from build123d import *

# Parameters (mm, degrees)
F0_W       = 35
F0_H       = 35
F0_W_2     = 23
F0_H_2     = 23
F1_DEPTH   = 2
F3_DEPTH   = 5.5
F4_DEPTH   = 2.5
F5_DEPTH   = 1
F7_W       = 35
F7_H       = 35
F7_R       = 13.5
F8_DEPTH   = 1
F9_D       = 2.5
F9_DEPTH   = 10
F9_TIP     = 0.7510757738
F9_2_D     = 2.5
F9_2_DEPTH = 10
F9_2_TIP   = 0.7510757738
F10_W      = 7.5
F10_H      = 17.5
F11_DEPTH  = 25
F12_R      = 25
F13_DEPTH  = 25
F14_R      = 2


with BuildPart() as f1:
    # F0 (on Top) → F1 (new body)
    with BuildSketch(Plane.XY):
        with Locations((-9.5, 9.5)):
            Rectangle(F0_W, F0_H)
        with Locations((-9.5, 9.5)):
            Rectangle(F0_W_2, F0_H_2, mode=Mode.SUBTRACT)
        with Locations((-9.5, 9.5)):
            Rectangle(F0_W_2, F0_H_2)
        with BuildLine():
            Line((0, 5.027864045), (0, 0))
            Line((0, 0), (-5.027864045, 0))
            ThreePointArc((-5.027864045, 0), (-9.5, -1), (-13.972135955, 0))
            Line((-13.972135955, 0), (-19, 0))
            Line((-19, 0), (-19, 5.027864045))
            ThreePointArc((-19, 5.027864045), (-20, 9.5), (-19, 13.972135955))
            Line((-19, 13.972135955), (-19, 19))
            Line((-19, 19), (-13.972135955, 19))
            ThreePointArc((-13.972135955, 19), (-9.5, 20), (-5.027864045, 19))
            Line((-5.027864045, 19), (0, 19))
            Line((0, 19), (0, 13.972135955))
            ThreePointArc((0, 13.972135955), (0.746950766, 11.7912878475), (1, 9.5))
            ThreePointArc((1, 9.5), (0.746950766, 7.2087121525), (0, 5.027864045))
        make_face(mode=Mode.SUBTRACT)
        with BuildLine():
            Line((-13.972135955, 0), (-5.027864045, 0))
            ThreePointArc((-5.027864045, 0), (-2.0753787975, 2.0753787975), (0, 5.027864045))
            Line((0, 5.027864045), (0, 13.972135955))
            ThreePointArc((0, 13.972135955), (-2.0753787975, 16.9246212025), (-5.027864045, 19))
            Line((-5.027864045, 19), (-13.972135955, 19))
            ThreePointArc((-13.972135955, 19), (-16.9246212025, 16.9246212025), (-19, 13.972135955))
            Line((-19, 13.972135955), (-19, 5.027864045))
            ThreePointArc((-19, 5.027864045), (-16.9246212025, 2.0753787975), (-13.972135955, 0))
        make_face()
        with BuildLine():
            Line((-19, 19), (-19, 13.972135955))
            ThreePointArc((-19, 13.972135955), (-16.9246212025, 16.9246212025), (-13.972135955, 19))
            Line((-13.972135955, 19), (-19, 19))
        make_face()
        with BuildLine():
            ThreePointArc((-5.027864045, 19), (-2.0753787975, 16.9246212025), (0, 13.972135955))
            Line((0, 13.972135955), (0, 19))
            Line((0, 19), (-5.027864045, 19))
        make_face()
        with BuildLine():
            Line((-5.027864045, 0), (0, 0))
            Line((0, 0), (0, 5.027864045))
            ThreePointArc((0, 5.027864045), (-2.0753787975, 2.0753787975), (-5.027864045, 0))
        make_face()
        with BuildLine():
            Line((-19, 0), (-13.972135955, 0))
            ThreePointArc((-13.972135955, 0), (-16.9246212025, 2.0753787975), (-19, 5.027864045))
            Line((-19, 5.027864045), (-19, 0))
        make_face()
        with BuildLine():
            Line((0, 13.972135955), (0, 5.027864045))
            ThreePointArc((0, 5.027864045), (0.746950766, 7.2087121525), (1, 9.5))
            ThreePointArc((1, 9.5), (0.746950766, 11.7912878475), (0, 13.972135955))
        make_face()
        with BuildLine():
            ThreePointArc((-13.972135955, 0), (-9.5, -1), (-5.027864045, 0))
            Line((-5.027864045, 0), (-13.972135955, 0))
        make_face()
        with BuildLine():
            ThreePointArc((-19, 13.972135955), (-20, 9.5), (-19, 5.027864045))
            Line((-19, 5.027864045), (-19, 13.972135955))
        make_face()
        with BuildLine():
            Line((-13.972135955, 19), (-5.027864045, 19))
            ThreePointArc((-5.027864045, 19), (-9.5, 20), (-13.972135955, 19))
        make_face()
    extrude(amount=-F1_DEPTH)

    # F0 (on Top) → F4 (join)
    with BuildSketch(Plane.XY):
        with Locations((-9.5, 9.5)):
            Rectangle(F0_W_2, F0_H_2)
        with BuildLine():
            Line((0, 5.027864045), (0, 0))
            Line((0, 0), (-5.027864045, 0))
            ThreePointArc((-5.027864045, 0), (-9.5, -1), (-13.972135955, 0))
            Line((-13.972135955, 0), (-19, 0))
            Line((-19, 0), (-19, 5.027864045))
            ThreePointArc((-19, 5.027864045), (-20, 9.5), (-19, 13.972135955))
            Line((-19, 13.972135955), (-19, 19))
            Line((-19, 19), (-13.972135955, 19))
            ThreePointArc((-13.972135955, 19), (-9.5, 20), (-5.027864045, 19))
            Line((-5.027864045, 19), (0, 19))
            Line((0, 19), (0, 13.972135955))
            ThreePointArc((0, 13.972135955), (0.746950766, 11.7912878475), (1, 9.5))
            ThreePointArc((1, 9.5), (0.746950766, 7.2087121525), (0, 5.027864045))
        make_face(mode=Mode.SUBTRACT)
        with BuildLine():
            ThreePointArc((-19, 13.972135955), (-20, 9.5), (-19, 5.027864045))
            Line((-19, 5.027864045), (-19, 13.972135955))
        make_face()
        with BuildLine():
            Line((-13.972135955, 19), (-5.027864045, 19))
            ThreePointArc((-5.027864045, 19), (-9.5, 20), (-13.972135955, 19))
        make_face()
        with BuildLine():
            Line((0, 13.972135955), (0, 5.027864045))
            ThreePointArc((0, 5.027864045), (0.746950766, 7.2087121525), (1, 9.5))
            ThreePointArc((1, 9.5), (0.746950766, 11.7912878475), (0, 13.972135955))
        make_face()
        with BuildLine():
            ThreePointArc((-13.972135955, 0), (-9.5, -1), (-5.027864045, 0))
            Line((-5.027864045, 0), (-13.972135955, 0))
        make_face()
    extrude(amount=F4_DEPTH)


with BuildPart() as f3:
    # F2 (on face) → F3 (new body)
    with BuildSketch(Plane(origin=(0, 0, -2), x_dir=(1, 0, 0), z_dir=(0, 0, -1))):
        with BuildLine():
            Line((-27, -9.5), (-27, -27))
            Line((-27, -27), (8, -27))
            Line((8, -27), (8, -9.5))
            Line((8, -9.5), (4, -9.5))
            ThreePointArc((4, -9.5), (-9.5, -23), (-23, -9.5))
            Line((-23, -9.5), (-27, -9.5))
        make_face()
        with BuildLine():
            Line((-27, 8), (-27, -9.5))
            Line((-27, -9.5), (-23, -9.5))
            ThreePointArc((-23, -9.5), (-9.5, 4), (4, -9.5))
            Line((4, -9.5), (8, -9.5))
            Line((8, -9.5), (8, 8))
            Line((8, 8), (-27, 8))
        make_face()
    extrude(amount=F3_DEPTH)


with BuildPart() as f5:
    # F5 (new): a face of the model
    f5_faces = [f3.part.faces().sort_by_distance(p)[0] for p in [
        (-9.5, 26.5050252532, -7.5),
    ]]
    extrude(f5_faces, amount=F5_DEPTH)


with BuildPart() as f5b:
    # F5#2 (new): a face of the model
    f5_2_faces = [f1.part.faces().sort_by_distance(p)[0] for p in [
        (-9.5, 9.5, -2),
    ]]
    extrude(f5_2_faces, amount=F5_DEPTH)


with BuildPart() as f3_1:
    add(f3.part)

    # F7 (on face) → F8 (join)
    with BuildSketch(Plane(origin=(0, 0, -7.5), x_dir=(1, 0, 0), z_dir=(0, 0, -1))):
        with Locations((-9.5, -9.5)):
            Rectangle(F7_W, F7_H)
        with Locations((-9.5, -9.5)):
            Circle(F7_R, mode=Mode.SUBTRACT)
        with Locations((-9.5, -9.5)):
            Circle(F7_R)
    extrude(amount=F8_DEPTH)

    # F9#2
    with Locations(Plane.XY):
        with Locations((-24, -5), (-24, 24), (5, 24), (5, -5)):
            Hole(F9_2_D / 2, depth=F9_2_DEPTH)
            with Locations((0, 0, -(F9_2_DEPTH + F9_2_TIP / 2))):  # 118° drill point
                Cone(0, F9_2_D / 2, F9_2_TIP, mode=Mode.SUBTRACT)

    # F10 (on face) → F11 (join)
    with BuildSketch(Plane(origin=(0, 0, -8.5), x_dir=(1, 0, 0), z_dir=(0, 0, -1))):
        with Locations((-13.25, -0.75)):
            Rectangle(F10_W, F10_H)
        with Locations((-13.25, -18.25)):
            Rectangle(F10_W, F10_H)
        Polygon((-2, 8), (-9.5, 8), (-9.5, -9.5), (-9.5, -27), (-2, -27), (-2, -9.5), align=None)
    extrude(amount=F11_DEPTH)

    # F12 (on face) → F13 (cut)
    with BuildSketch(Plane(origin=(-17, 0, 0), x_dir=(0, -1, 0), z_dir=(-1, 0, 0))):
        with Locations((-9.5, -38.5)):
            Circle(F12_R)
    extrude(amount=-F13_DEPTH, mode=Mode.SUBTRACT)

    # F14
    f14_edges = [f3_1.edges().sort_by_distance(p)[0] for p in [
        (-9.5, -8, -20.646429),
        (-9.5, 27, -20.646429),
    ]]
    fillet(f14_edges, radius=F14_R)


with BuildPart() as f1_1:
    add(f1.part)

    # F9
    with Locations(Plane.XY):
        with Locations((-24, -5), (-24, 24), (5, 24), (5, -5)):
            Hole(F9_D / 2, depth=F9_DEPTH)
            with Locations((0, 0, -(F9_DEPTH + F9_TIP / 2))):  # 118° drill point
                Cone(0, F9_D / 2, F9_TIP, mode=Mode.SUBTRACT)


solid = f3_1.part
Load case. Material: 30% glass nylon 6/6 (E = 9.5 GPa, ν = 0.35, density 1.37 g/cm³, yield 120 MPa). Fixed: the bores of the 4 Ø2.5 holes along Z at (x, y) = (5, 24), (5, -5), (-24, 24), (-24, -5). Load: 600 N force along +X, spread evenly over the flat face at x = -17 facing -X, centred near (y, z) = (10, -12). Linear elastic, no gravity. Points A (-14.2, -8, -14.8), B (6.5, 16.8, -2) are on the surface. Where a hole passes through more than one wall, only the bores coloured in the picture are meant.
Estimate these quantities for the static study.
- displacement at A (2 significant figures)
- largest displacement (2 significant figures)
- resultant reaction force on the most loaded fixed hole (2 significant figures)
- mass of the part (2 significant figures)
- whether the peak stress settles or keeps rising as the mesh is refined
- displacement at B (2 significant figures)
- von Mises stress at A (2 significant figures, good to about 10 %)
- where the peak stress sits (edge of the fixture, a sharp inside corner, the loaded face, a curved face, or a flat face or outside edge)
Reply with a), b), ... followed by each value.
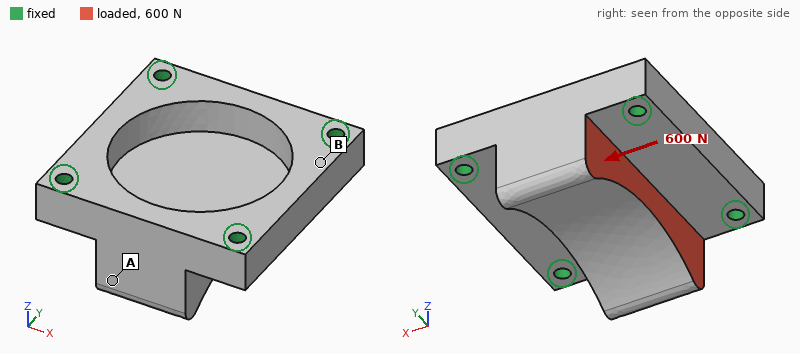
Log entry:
a) 12 µm
b) 16 µm
c) 180 N
d) 11 g
e) keeps rising
f) 3.3 µm
g) 2.5 MPa
h) edge of the fixture
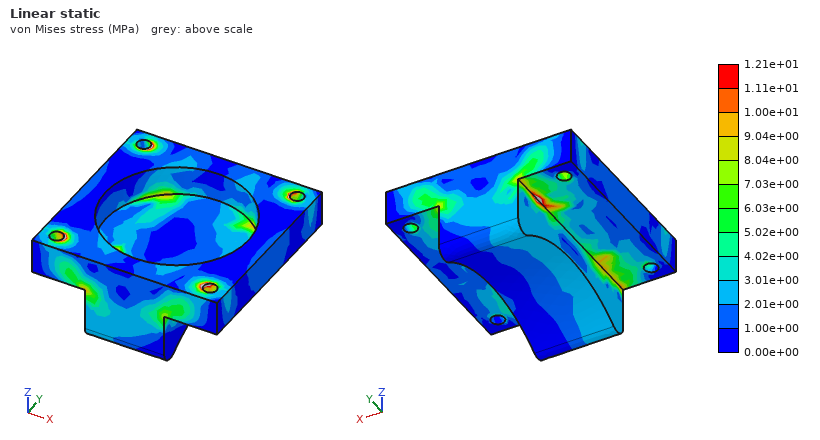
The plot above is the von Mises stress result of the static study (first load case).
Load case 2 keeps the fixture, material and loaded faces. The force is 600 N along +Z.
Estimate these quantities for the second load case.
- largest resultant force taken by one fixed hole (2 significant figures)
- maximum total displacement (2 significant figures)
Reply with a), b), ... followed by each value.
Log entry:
a) 270 N
b) 50 µm
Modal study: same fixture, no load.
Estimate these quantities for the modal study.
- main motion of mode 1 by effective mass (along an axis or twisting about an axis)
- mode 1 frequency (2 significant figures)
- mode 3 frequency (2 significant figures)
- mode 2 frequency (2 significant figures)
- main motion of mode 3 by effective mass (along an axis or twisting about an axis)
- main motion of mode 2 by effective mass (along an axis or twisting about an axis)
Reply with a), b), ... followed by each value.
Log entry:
a) along Z
b) 10 kHz
c) 14 kHz
d) 12 kHz
e) along Y
f) along Y
